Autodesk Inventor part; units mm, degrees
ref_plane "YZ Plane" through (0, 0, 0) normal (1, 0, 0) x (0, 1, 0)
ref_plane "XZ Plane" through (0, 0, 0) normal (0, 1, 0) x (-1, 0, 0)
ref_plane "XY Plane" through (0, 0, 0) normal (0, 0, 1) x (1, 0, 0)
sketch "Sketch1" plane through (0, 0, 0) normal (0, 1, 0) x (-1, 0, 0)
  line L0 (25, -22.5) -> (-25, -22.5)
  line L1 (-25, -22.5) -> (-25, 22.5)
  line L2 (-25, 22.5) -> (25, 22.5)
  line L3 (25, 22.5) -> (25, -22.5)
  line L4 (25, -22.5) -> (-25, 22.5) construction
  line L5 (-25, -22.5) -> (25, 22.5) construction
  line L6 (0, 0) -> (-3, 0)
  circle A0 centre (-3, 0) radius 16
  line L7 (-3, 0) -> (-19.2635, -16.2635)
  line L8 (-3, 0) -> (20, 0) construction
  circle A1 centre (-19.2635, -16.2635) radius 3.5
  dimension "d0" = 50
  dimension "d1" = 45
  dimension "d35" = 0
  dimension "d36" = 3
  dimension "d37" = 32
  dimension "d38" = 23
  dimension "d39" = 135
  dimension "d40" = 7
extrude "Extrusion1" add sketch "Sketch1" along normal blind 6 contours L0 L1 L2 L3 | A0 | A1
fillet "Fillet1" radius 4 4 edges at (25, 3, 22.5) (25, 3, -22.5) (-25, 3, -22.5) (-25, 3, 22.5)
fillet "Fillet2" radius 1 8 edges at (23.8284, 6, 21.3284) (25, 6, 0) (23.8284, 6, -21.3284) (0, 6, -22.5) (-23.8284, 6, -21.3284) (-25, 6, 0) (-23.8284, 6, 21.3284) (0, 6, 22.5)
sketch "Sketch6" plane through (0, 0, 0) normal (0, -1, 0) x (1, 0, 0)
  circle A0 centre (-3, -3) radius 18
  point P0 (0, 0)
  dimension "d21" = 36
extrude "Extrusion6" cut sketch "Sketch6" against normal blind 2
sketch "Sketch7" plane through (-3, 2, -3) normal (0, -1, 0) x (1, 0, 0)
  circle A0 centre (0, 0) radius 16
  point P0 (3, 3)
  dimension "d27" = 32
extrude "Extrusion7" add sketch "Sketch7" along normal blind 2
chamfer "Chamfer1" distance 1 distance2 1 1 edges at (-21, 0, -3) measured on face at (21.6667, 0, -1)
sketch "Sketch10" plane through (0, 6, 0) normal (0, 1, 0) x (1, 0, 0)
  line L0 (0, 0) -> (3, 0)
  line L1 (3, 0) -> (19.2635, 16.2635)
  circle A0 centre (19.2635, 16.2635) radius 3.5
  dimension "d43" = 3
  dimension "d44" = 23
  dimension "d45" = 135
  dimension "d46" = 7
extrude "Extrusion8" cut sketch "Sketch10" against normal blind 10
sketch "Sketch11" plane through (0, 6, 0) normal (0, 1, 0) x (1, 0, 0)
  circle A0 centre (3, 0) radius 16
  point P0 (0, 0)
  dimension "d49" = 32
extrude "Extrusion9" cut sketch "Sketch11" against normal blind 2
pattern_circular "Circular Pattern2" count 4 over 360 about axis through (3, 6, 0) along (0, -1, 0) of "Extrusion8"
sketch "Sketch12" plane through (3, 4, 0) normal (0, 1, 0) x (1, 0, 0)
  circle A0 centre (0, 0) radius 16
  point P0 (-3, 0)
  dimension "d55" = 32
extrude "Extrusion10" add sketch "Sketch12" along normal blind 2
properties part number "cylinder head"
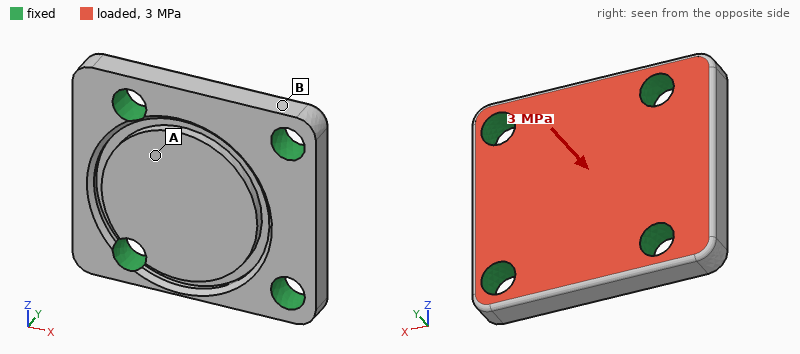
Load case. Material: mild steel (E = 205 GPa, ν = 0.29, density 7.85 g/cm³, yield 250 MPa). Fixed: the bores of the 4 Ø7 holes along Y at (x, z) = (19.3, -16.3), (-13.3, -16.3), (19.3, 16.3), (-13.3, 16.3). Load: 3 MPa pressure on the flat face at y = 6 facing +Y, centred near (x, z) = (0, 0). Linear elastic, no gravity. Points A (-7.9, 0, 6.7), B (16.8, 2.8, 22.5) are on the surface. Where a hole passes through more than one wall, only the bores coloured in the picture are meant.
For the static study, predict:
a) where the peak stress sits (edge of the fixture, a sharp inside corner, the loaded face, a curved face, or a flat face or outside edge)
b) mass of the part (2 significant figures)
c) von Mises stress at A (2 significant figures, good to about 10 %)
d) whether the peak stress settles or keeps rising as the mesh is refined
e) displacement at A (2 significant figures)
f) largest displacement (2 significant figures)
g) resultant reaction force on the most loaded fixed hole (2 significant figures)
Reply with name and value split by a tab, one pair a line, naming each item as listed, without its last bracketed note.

where the peak stress sits	edge of the fixture
mass of the part	94 g
von Mises stress at A	17 MPa
whether the peak stress settles or keeps rising as the mesh is refined	keeps rising
displacement at A	3.2 µm
largest displacement	5.0 µm
resultant reaction force on the most loaded fixed hole	1.7 kN
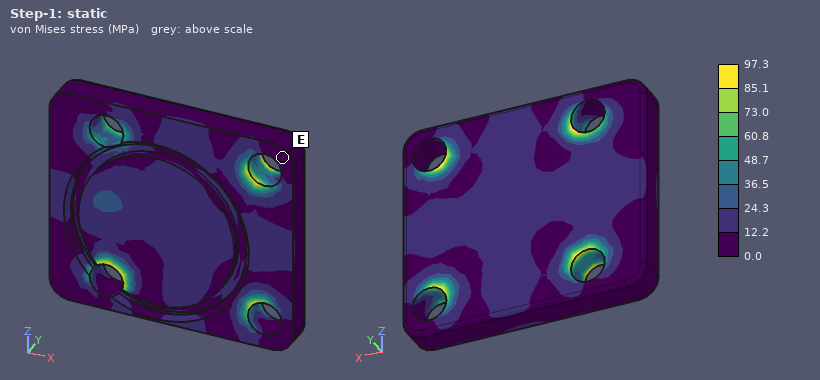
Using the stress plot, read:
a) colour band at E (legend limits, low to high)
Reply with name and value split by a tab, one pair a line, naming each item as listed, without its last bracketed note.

colour band at E	0.0 to 12.2 MPa
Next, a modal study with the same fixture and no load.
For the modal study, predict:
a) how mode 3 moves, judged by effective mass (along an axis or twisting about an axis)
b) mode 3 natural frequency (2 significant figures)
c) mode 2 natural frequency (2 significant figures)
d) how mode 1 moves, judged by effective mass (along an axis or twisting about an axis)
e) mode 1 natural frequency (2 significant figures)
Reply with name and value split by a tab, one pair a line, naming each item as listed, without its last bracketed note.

how mode 3 moves, judged by effective mass	twisting about X
mode 3 natural frequency	33 kHz
mode 2 natural frequency	25 kHz
how mode 1 moves, judged by effective mass	along Y
mode 1 natural frequency	22 kHz
